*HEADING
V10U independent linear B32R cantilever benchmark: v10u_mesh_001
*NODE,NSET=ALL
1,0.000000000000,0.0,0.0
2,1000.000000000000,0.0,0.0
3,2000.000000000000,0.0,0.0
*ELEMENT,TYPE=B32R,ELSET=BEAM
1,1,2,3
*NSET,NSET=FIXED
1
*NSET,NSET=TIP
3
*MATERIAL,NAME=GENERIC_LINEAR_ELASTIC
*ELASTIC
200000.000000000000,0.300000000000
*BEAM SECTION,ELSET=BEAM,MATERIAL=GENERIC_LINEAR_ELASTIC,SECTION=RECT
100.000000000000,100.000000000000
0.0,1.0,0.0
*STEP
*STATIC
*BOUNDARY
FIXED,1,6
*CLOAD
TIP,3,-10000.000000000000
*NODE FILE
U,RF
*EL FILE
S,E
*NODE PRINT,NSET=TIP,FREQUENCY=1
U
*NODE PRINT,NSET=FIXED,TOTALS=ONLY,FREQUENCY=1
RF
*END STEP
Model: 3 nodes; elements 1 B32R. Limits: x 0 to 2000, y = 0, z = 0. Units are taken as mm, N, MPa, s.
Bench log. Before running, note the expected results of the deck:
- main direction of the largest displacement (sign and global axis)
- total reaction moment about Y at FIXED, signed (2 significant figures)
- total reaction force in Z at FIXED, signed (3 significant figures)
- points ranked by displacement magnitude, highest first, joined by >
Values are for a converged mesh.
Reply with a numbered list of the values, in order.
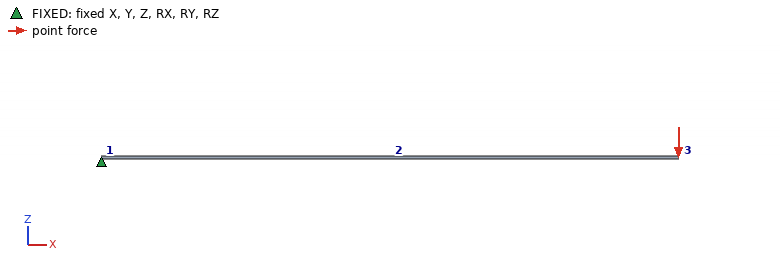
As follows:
1. -Z
2. -2.0e+07 N·mm
3. 10000 N
4. node 3 > node 2 > node 1
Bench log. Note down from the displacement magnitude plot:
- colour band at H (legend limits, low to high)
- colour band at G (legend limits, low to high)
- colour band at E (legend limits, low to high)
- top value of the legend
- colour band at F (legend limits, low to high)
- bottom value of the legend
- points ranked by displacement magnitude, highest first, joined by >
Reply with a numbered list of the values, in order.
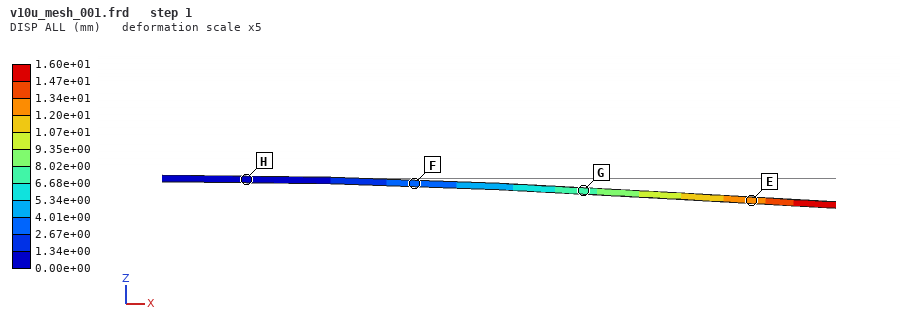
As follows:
1. 0.00e+00 to 1.34e+00 mm
2. 6.68e+00 to 8.02e+00 mm
3. 1.20e+01 to 1.34e+01 mm
4. 1.60e+01 mm
5. 2.67e+00 to 4.01e+00 mm
6. 0.00e+00 mm
7. E > G > F > H
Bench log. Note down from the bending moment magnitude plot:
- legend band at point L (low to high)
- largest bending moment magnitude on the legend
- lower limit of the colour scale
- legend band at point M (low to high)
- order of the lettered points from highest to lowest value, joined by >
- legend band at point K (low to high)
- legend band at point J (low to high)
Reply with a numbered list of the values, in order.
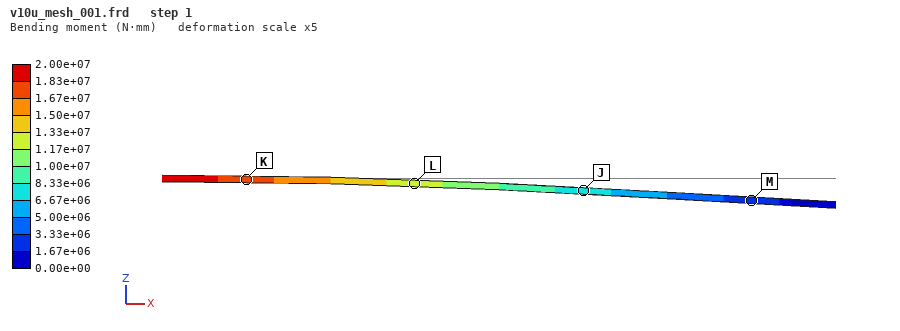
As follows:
1. 1.17e+07 to 1.33e+07 N·mm
2. 2.00e+07 N·mm
3. 0.00e+00 N·mm
4. 1.67e+06 to 3.33e+06 N·mm
5. K > L > J > M
6. 1.67e+07 to 1.83e+07 N·mm
7. 6.67e+06 to 8.33e+06 N·mm
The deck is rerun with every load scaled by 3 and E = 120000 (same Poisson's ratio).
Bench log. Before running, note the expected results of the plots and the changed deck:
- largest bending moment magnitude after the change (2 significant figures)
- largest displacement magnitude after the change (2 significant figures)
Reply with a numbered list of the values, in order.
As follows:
1. 6.0e+07 N·mm
2. 80 mm
